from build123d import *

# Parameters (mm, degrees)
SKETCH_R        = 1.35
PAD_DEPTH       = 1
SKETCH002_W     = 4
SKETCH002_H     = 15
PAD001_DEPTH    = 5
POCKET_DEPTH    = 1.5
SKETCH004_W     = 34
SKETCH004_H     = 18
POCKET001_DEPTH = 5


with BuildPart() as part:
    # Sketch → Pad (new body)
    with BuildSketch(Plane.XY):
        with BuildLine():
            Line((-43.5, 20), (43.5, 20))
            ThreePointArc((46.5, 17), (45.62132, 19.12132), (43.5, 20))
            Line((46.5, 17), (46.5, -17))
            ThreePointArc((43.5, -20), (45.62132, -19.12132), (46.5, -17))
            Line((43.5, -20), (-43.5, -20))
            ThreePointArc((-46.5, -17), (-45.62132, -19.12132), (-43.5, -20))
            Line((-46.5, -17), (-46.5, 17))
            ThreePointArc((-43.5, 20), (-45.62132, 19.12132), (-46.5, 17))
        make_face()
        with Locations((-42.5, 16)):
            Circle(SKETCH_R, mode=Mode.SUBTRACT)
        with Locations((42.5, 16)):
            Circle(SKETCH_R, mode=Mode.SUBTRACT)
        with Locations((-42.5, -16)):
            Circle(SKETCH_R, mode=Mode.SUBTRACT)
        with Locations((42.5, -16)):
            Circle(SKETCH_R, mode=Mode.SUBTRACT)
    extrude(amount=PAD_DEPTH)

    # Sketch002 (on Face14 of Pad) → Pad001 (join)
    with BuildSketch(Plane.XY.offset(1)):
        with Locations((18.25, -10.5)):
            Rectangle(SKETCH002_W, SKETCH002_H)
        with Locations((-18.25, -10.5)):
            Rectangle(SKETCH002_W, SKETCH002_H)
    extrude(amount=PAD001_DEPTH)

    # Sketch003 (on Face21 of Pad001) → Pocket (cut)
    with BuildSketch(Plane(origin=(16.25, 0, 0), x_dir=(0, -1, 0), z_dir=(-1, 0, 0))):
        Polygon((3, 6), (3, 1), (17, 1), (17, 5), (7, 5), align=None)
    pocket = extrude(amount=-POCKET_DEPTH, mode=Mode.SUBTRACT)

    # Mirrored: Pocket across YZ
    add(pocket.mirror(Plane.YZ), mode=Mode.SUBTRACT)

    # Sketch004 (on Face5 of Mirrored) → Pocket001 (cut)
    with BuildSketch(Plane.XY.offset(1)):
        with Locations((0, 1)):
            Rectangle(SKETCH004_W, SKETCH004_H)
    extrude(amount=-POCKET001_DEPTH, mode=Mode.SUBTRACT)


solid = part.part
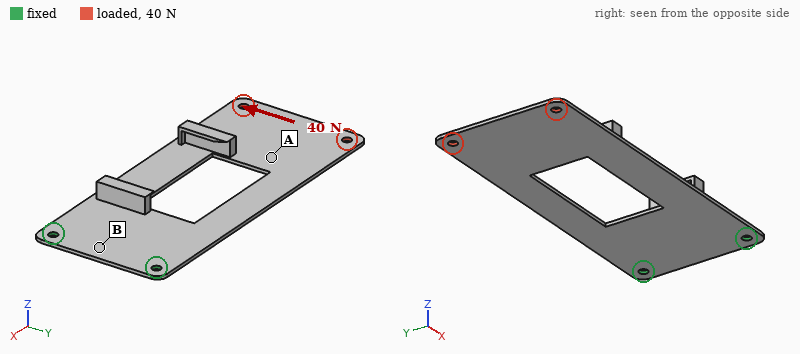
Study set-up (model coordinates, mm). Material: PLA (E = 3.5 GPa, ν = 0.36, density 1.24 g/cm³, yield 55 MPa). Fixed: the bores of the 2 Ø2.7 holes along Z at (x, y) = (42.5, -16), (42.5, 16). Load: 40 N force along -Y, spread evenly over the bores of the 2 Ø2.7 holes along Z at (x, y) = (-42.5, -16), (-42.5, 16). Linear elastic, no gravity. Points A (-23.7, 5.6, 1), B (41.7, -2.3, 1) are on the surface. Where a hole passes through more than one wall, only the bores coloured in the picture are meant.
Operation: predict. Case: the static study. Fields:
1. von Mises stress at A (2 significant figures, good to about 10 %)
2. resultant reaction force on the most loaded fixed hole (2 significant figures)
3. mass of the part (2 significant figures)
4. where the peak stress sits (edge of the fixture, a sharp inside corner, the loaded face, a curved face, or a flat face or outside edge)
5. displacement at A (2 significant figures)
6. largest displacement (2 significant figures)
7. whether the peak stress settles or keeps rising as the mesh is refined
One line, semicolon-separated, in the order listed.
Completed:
5.8 MPa; 110 N; 4.3 g; a sharp inside corner; 0.78 mm; 1.0 mm; keeps rising
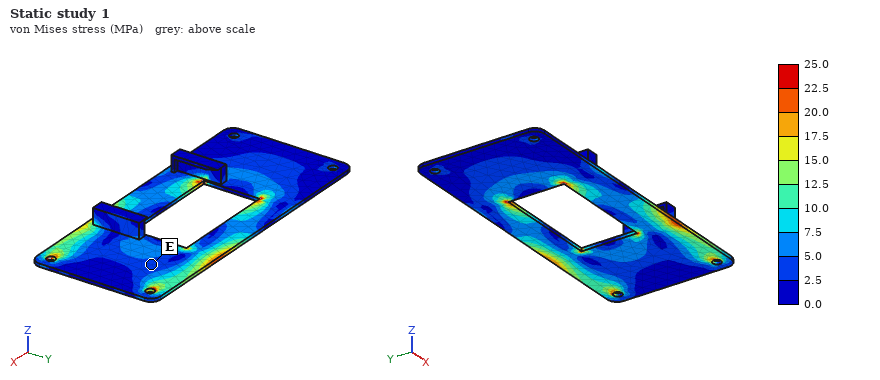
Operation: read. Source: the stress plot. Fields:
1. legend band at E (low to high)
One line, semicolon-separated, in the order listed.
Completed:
2.5 to 5.0 MPa
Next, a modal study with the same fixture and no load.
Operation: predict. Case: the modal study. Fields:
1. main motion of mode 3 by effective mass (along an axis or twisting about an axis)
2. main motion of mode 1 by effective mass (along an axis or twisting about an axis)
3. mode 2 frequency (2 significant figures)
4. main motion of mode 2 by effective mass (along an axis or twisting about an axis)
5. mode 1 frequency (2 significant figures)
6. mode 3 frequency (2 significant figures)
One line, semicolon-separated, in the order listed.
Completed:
along Z; along Z; 150 Hz; twisting about X; 31 Hz; 200 Hz
